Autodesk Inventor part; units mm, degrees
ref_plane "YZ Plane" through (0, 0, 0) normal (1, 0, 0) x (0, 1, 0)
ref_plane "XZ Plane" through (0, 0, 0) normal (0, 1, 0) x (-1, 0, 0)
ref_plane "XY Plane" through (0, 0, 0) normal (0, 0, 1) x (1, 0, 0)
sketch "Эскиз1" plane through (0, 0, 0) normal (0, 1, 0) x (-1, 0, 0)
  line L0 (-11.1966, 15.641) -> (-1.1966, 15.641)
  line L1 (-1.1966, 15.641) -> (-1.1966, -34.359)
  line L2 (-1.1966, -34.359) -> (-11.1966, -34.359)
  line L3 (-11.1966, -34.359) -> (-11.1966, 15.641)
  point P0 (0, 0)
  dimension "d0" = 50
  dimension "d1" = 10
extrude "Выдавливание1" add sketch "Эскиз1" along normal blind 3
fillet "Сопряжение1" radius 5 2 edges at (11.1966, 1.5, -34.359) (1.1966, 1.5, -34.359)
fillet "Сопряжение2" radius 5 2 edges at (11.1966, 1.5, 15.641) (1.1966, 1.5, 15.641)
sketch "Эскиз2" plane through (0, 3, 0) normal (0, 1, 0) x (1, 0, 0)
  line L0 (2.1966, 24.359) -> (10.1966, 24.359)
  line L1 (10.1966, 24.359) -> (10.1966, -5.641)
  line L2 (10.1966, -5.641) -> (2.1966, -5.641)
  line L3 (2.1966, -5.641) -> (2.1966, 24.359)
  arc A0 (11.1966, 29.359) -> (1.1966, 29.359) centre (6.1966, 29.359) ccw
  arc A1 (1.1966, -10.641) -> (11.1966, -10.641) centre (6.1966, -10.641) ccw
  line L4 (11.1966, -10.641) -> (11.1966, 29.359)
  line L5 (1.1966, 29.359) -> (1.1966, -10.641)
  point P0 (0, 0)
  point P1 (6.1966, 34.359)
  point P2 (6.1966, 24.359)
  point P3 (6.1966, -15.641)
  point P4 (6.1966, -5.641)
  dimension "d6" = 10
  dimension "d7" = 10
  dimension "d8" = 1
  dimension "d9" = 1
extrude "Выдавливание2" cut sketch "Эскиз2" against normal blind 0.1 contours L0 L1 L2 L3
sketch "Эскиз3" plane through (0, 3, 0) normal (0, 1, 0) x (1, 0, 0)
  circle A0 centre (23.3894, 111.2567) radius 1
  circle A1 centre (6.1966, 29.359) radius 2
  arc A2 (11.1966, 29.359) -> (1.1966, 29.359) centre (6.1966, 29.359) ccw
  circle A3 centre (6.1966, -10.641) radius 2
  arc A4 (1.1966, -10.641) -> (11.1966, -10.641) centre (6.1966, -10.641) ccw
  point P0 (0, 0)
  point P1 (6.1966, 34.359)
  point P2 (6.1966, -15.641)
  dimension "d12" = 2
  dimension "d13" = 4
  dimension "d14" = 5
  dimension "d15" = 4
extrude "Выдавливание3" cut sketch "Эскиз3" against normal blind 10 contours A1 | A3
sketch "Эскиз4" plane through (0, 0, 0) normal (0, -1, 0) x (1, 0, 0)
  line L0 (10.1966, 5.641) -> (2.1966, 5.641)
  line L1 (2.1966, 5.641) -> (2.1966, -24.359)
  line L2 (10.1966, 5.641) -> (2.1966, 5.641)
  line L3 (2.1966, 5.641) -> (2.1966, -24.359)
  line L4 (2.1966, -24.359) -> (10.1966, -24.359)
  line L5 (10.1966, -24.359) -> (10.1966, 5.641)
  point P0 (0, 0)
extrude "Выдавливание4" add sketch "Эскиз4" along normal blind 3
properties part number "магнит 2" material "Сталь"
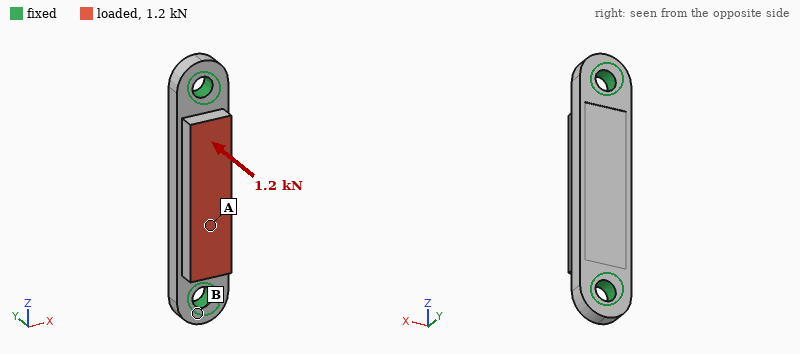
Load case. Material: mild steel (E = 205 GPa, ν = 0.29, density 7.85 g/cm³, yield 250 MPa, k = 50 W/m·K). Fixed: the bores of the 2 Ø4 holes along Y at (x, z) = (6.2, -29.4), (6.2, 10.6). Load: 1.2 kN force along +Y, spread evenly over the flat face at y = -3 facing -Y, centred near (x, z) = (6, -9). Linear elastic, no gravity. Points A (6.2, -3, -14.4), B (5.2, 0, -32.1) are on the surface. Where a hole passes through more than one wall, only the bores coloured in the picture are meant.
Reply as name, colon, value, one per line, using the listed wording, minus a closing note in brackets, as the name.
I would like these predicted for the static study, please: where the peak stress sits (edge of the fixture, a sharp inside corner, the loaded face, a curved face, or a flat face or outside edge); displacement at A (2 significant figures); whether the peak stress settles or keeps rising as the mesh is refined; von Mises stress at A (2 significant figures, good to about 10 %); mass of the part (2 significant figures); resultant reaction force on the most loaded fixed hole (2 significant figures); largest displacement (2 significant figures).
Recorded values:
where the peak stress sits: edge of the fixture
displacement at A: 13 µm
whether the peak stress settles or keeps rising as the mesh is refined: keeps rising
von Mises stress at A: 71 MPa
mass of the part: 16 g
resultant reaction force on the most loaded fixed hole: 870 N
largest displacement: 15 µm
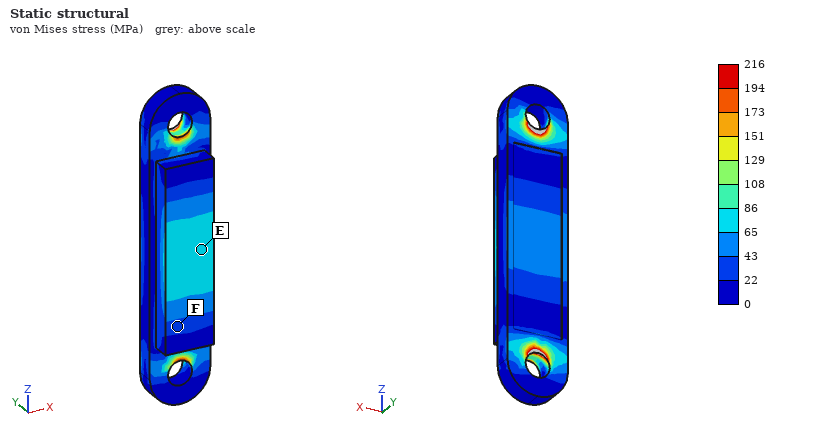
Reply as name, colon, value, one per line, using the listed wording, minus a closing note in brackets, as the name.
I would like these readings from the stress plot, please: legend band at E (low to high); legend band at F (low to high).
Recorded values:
legend band at E: 65 to 86 MPa
legend band at F: 22 to 43 MPa
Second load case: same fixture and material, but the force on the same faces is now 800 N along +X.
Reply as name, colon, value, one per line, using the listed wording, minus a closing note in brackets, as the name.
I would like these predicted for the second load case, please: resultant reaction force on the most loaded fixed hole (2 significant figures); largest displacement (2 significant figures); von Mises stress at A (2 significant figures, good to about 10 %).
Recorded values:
resultant reaction force on the most loaded fixed hole: 400 N
largest displacement: 12 µm
von Mises stress at A: 18 MPa
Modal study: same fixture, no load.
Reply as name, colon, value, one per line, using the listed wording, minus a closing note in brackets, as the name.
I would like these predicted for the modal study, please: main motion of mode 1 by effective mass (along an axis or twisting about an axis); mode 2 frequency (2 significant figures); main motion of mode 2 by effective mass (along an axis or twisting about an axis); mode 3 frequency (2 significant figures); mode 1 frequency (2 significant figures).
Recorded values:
main motion of mode 1 by effective mass: along Y
mode 2 frequency: 18 kHz
main motion of mode 2 by effective mass: along X
mode 3 frequency: 24 kHz
mode 1 frequency: 14 kHz
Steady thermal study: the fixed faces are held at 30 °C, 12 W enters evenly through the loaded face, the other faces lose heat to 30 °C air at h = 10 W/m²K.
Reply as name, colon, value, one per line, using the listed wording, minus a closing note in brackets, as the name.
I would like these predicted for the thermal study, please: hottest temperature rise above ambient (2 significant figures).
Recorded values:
hottest temperature rise above ambient: 38 K
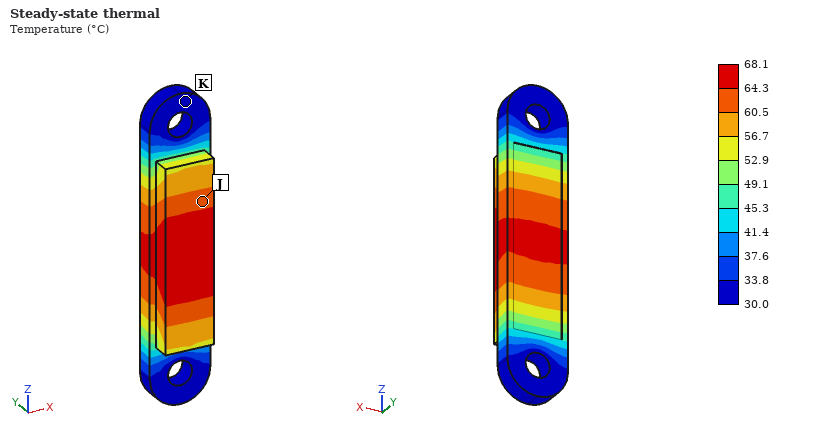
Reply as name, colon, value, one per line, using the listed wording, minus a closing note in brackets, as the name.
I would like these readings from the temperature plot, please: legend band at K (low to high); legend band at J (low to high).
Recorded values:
legend band at K: 30.0 to 33.8 °C
legend band at J: 60.5 to 64.3 °C
